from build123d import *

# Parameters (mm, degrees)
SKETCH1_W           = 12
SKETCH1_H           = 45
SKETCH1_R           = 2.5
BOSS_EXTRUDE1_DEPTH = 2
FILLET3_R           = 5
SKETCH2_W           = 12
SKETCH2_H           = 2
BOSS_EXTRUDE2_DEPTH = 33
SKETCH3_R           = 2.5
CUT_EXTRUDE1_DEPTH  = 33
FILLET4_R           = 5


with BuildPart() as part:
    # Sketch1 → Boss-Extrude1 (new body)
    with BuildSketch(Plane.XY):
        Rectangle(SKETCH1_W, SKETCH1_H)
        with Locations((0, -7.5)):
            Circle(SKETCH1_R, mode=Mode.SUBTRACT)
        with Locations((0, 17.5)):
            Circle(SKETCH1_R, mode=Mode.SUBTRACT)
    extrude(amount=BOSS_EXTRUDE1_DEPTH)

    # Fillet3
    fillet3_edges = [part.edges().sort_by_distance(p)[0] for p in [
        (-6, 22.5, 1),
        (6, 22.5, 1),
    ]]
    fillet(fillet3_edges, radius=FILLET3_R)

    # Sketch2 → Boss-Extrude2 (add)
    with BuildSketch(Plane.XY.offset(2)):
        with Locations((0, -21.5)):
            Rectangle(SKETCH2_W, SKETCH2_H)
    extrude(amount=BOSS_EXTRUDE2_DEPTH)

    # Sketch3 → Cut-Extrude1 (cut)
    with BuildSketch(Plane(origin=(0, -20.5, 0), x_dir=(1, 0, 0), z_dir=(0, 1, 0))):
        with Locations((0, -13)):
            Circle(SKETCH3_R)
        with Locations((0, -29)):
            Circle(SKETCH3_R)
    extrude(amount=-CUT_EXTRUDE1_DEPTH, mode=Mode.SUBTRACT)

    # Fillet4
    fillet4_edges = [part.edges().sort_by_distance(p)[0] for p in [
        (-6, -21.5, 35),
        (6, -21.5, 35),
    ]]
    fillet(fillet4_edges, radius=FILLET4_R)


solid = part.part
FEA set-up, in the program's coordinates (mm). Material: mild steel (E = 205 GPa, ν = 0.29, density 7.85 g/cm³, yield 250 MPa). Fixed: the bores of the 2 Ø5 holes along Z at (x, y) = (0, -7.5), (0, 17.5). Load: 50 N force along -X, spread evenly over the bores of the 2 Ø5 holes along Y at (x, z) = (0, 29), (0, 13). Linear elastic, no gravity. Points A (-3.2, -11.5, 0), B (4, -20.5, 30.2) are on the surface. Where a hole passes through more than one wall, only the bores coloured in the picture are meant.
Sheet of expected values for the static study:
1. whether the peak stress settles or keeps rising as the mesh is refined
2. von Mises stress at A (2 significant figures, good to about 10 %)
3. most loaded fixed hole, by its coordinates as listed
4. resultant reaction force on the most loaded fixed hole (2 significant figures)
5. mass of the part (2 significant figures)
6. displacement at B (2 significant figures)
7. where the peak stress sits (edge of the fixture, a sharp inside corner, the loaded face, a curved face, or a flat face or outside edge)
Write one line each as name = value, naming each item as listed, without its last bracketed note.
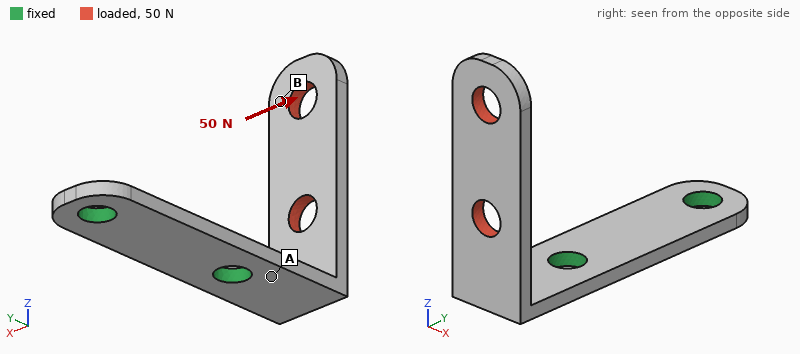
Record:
whether the peak stress settles or keeps rising as the mesh is refined = keeps rising
von Mises stress at A = 82 MPa
most loaded fixed hole, by its coordinates as listed = (0, -7.5)
resultant reaction force on the most loaded fixed hole = 58 N
mass of the part = 13 g
displacement at B = 0.13 mm
where the peak stress sits = edge of the fixture
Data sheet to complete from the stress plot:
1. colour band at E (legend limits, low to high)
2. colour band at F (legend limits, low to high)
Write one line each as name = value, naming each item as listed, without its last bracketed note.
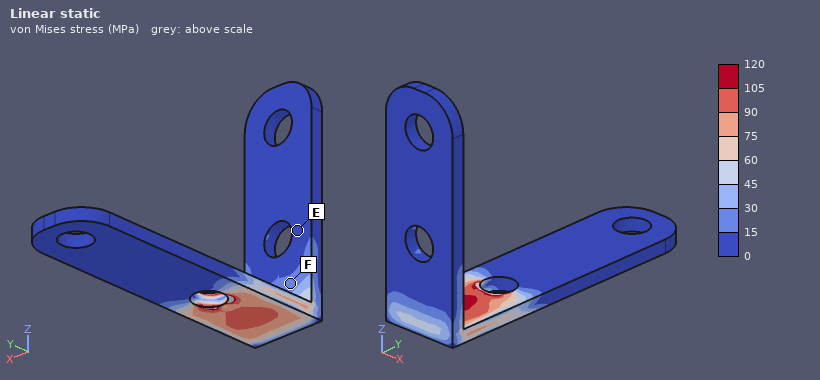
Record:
colour band at E = 0 to 15 MPa
colour band at F = 15 to 30 MPa
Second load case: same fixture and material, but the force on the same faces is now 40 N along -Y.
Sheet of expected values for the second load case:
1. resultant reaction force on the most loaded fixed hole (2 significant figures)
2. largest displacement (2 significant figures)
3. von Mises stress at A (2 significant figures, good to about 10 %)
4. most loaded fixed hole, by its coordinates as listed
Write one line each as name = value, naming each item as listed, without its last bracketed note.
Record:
resultant reaction force on the most loaded fixed hole = 39 N
largest displacement = 0.35 mm
von Mises stress at A = 86 MPa
most loaded fixed hole, by its coordinates as listed = (0, -7.5)
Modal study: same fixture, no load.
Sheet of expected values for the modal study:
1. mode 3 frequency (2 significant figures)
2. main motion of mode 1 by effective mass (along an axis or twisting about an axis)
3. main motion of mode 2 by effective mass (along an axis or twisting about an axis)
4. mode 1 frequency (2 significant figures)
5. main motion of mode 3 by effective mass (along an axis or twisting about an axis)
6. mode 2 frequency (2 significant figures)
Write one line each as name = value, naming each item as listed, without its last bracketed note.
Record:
mode 3 frequency = 4200 Hz
main motion of mode 1 by effective mass = along Y
main motion of mode 2 by effective mass = along X
mode 1 frequency = 1000 Hz
main motion of mode 3 by effective mass = along Z
mode 2 frequency = 1700 Hz
